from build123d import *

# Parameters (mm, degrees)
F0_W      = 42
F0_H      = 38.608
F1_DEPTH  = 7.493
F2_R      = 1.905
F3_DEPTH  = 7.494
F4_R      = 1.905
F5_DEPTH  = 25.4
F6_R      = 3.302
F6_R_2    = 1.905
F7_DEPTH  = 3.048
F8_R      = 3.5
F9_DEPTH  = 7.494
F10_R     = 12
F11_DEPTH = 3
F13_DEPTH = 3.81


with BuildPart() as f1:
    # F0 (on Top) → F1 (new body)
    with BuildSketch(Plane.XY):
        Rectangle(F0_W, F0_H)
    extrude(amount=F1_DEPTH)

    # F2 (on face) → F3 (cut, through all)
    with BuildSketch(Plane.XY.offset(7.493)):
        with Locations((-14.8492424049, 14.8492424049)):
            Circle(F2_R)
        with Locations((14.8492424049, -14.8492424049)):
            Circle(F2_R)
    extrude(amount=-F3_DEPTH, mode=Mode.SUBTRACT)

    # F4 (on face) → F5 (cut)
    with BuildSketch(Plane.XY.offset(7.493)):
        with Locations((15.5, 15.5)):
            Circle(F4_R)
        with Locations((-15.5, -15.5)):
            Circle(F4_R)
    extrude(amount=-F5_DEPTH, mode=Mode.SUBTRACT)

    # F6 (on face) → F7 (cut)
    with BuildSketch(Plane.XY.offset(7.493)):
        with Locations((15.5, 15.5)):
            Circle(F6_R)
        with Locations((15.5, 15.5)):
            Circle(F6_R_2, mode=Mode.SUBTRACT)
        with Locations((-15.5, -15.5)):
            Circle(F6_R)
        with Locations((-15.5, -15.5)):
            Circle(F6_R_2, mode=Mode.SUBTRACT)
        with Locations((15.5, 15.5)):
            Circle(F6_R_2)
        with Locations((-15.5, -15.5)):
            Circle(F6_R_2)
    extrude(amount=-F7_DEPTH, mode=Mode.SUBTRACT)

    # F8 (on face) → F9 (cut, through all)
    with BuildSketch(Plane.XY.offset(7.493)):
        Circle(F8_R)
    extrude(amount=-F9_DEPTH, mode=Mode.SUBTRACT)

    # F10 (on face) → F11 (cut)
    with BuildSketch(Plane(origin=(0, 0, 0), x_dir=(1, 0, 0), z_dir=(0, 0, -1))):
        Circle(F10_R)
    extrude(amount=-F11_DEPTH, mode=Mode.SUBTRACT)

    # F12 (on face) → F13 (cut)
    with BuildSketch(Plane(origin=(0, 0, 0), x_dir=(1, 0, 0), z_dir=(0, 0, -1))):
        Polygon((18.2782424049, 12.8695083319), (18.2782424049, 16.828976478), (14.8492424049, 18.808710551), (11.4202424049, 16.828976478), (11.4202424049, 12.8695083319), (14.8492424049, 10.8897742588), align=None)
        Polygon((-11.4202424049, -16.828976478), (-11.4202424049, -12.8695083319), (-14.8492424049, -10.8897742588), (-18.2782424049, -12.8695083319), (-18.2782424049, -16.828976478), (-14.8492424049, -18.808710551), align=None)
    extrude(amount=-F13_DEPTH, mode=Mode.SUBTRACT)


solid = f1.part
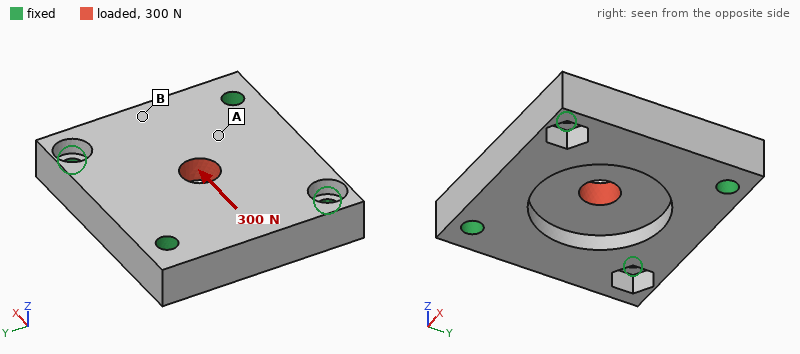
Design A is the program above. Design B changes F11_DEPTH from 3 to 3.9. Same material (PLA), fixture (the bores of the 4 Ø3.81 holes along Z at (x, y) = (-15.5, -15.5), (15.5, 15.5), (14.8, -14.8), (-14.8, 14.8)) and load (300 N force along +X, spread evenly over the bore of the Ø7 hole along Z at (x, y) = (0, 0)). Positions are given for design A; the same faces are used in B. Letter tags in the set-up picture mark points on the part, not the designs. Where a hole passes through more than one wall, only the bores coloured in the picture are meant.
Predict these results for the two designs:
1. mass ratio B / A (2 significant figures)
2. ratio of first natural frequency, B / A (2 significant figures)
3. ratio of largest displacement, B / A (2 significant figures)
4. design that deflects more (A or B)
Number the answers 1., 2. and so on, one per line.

1. 0.96
2. 1.0
3. 1.2
4. B
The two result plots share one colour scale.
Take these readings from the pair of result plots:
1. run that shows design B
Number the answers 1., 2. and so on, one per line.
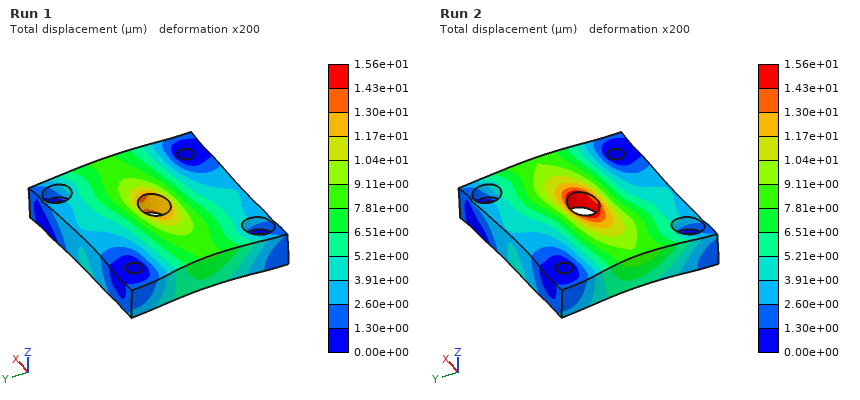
1. Run 2
